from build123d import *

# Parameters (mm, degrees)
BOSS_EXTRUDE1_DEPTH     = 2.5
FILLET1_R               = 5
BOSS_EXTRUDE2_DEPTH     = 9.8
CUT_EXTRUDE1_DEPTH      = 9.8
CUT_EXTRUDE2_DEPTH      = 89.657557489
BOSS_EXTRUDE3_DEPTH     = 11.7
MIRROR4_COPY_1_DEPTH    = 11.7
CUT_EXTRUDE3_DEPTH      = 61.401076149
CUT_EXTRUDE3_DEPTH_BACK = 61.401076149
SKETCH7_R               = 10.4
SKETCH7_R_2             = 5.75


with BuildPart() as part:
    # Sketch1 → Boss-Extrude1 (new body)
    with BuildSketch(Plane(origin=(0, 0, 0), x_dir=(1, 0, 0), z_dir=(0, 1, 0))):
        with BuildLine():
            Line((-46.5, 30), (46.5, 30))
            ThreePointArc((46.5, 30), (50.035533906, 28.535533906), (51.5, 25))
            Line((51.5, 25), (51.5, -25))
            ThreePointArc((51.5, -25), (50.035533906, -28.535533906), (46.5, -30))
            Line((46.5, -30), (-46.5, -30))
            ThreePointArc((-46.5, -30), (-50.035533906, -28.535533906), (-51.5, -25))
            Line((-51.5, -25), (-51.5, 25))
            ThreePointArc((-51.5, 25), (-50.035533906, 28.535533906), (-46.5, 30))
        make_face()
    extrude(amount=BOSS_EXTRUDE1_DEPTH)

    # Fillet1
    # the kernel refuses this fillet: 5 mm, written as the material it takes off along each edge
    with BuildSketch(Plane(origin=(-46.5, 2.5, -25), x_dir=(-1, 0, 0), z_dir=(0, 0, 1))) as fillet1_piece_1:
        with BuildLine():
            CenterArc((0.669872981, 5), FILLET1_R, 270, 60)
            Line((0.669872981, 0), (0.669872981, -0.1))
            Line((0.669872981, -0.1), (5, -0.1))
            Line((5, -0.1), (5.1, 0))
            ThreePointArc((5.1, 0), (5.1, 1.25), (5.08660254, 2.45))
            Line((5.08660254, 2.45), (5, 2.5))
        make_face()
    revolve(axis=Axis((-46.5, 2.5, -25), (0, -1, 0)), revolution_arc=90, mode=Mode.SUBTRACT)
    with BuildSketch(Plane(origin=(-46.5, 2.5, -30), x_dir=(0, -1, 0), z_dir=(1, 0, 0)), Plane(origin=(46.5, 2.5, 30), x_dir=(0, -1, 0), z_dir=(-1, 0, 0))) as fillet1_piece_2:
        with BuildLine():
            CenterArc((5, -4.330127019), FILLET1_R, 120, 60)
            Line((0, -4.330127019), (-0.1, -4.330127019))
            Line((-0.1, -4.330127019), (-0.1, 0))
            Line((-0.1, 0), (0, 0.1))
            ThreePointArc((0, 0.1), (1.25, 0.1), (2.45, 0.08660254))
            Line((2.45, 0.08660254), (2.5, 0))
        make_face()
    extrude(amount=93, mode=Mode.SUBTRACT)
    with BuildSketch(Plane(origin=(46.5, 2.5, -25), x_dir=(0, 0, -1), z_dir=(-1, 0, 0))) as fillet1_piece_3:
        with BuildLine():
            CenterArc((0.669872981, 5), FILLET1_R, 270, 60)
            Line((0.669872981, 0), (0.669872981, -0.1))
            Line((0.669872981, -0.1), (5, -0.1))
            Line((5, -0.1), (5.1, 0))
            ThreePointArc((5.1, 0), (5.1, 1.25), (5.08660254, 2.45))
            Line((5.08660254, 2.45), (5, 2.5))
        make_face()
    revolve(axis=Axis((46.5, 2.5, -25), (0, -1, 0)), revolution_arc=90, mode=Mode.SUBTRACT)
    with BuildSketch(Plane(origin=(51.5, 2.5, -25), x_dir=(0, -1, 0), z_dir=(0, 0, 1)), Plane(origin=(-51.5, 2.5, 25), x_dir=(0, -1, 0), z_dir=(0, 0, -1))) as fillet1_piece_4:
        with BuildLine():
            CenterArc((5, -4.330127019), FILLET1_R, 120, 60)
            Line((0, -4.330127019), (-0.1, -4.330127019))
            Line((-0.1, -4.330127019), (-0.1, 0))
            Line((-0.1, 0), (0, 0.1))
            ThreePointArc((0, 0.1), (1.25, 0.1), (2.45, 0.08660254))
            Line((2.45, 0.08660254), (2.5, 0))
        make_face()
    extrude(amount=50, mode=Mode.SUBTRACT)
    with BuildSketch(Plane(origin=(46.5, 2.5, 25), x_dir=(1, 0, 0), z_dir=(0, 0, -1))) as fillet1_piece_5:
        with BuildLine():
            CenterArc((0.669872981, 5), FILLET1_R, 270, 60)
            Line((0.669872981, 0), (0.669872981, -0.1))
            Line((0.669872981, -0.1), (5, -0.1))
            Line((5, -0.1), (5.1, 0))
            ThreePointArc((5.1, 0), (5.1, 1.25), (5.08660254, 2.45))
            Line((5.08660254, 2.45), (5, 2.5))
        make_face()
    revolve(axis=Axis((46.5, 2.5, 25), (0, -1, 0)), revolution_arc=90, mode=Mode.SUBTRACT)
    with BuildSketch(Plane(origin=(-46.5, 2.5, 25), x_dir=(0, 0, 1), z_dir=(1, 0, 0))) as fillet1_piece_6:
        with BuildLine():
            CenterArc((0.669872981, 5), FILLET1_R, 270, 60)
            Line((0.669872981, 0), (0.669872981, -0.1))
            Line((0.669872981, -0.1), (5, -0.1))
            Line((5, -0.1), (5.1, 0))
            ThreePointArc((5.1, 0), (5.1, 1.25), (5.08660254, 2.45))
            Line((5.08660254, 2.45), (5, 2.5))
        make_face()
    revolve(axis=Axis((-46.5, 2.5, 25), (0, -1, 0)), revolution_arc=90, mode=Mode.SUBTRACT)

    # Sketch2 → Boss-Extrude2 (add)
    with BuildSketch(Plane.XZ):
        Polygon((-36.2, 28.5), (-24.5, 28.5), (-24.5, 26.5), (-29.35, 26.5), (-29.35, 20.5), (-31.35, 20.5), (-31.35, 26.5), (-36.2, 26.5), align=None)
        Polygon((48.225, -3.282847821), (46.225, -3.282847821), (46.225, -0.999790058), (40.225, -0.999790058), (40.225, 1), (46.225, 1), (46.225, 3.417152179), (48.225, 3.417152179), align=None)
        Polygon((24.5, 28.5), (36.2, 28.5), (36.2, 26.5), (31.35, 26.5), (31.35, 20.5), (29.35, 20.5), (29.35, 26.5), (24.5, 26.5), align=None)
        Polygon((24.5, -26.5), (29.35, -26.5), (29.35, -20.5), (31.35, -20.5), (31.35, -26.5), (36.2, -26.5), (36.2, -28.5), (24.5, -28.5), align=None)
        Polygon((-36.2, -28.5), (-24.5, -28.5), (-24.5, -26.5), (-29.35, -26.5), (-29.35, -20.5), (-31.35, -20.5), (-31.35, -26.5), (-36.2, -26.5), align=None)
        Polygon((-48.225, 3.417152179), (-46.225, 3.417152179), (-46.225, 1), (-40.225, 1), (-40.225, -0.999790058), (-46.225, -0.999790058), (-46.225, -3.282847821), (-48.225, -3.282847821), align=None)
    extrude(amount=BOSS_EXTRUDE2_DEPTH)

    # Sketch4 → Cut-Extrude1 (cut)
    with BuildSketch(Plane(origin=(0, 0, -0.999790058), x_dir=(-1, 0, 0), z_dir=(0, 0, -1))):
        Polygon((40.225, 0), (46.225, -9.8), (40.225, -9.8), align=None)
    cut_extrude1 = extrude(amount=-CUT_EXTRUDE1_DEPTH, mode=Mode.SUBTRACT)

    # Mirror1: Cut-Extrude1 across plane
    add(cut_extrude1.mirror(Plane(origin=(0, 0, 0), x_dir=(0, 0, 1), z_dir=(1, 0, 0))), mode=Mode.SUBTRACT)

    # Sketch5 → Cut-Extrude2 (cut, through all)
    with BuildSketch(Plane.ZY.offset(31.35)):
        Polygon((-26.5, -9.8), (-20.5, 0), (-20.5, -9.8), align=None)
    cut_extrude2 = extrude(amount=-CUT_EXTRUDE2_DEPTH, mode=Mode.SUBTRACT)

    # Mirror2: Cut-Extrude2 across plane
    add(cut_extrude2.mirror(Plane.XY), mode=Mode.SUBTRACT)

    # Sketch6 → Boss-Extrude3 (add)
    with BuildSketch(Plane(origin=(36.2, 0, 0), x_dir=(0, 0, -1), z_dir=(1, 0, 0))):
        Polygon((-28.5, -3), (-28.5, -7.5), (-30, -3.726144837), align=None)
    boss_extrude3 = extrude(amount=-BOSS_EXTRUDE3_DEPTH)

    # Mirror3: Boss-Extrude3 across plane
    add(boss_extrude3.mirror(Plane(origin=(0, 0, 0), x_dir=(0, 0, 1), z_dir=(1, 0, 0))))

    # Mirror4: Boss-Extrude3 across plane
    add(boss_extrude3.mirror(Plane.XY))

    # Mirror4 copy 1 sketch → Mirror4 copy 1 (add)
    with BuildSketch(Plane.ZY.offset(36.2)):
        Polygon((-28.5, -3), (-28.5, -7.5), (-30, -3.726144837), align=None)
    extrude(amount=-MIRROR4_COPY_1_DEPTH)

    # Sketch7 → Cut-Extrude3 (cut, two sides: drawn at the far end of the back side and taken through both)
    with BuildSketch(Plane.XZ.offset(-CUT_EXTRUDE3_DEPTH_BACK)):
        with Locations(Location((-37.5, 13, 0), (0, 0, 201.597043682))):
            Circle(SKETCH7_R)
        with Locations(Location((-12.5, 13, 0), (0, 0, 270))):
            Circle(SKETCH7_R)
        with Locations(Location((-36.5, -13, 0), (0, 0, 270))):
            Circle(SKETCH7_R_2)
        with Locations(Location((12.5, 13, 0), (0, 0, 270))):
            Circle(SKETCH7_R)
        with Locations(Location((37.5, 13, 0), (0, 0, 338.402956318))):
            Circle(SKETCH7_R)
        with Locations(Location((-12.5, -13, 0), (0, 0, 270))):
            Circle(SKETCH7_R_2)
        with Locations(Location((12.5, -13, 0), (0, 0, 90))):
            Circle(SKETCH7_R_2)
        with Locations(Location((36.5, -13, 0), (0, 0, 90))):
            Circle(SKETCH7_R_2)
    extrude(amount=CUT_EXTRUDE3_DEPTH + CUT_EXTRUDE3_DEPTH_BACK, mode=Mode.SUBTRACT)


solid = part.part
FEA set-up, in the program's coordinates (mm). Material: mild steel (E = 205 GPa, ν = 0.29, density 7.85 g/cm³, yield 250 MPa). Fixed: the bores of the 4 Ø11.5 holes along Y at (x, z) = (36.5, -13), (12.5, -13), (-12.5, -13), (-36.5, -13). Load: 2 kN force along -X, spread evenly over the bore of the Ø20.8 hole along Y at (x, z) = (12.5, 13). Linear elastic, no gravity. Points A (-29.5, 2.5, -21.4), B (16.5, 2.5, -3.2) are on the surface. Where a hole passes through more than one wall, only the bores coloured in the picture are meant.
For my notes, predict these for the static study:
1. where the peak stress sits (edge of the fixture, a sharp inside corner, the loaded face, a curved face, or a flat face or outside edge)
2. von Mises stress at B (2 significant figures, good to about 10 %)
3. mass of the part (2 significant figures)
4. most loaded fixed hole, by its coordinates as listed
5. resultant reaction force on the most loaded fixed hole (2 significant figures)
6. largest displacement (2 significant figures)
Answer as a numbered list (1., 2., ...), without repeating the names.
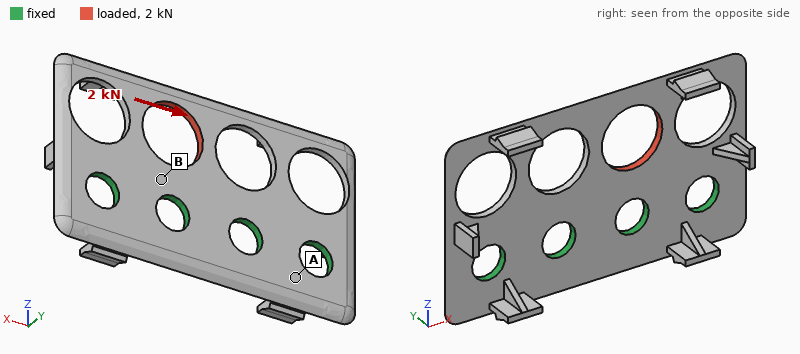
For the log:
1. the loaded face
2. 34 MPa
3. 92 g
4. (36.5, -13)
5. 850 N
6. 21 µm
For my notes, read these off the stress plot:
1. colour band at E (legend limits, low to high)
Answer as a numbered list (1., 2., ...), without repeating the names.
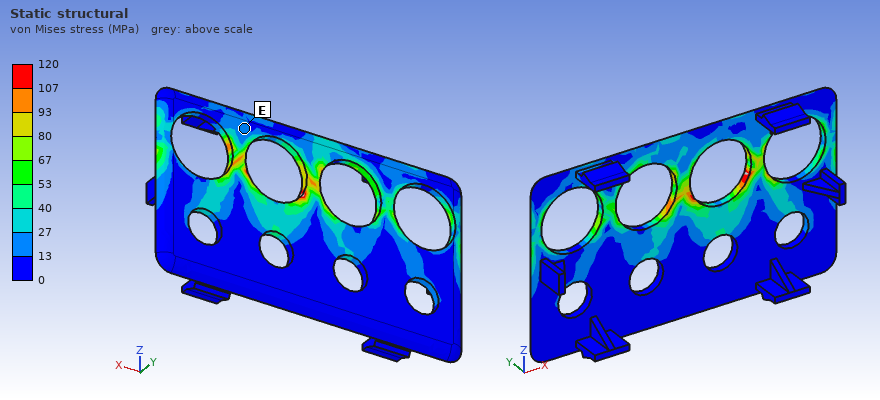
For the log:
1. 13 to 27 MPa
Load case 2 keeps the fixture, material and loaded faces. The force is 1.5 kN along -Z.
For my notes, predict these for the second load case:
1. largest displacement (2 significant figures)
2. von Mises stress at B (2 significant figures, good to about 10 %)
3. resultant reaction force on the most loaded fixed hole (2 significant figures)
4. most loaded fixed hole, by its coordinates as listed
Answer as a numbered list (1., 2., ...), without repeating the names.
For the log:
1. 7.0 µm
2. 13 MPa
3. 750 N
4. (12.5, -13)
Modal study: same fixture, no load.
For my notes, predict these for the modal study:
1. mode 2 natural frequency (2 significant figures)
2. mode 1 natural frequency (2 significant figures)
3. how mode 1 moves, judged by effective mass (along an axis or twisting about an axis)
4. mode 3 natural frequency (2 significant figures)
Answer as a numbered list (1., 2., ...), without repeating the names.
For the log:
1. 1500 Hz
2. 1100 Hz
3. along Y
4. 2600 Hz
